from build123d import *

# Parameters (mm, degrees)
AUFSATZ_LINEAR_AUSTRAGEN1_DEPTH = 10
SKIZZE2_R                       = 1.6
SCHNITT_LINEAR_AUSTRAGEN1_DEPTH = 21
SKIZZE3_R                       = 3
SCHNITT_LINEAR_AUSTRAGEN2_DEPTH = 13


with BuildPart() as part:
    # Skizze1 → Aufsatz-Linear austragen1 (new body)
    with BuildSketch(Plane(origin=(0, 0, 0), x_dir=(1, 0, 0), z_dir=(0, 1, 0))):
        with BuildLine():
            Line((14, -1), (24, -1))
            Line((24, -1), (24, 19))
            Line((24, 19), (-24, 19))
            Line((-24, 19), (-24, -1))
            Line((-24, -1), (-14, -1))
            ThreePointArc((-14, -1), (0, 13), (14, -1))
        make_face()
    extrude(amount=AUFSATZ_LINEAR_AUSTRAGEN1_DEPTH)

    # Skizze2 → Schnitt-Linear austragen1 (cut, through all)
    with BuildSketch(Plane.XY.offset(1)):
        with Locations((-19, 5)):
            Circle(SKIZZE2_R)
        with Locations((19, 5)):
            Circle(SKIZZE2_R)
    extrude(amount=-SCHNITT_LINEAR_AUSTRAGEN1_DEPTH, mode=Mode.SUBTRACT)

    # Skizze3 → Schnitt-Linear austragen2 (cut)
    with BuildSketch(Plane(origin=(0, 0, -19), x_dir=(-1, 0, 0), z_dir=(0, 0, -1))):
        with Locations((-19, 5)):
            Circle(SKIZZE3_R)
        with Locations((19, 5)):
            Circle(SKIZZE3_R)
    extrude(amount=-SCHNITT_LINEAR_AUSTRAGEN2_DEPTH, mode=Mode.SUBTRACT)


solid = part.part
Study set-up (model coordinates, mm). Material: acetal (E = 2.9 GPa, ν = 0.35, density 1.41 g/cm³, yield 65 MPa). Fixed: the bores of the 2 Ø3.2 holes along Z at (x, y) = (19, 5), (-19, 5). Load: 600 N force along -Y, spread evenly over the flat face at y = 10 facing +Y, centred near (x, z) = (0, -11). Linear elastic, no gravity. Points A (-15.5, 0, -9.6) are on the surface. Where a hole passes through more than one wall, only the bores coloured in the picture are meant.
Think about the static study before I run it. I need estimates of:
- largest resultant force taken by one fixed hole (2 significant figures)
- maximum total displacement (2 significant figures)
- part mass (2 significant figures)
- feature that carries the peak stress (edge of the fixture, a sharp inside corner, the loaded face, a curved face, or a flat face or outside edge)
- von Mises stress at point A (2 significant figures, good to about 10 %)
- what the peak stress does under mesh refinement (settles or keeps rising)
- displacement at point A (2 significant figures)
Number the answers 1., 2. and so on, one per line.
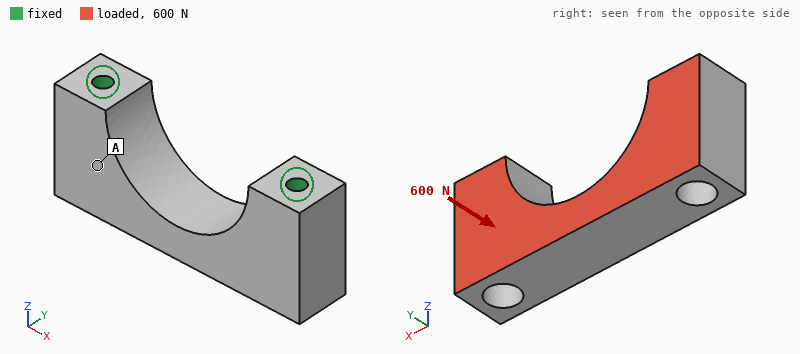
1. 300 N
2. 0.25 mm
3. 8.0 g
4. edge of the fixture
5. 4.3 MPa
6. keeps rising
7. 0.100 mm
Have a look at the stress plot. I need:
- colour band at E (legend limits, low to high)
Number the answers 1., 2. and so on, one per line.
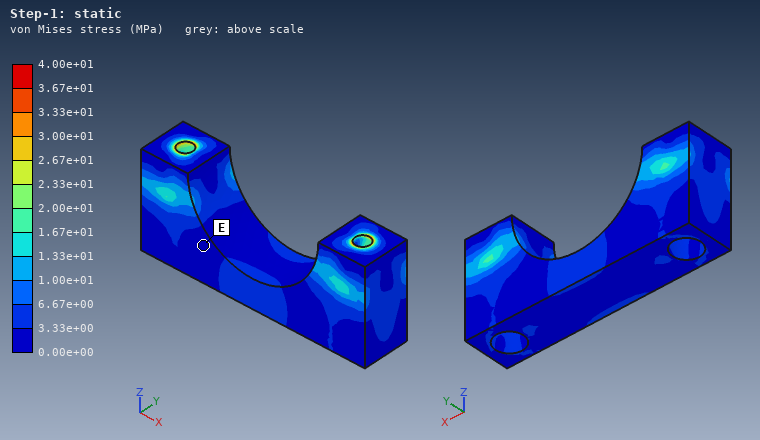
1. 0.00e+00 to 3.33e+00 MPa
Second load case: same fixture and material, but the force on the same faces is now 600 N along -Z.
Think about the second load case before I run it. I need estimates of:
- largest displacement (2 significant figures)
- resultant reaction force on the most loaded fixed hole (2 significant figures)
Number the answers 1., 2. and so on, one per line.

1. 0.14 mm
2. 310 N
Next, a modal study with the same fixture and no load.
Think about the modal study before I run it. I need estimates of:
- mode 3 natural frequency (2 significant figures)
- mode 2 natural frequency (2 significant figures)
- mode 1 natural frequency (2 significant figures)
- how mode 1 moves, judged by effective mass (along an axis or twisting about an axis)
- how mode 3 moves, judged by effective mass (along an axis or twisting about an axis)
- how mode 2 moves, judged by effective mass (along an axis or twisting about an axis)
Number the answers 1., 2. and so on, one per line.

1. 6100 Hz
2. 5700 Hz
3. 3300 Hz
4. along Y
5. along X
6. twisting about Z
